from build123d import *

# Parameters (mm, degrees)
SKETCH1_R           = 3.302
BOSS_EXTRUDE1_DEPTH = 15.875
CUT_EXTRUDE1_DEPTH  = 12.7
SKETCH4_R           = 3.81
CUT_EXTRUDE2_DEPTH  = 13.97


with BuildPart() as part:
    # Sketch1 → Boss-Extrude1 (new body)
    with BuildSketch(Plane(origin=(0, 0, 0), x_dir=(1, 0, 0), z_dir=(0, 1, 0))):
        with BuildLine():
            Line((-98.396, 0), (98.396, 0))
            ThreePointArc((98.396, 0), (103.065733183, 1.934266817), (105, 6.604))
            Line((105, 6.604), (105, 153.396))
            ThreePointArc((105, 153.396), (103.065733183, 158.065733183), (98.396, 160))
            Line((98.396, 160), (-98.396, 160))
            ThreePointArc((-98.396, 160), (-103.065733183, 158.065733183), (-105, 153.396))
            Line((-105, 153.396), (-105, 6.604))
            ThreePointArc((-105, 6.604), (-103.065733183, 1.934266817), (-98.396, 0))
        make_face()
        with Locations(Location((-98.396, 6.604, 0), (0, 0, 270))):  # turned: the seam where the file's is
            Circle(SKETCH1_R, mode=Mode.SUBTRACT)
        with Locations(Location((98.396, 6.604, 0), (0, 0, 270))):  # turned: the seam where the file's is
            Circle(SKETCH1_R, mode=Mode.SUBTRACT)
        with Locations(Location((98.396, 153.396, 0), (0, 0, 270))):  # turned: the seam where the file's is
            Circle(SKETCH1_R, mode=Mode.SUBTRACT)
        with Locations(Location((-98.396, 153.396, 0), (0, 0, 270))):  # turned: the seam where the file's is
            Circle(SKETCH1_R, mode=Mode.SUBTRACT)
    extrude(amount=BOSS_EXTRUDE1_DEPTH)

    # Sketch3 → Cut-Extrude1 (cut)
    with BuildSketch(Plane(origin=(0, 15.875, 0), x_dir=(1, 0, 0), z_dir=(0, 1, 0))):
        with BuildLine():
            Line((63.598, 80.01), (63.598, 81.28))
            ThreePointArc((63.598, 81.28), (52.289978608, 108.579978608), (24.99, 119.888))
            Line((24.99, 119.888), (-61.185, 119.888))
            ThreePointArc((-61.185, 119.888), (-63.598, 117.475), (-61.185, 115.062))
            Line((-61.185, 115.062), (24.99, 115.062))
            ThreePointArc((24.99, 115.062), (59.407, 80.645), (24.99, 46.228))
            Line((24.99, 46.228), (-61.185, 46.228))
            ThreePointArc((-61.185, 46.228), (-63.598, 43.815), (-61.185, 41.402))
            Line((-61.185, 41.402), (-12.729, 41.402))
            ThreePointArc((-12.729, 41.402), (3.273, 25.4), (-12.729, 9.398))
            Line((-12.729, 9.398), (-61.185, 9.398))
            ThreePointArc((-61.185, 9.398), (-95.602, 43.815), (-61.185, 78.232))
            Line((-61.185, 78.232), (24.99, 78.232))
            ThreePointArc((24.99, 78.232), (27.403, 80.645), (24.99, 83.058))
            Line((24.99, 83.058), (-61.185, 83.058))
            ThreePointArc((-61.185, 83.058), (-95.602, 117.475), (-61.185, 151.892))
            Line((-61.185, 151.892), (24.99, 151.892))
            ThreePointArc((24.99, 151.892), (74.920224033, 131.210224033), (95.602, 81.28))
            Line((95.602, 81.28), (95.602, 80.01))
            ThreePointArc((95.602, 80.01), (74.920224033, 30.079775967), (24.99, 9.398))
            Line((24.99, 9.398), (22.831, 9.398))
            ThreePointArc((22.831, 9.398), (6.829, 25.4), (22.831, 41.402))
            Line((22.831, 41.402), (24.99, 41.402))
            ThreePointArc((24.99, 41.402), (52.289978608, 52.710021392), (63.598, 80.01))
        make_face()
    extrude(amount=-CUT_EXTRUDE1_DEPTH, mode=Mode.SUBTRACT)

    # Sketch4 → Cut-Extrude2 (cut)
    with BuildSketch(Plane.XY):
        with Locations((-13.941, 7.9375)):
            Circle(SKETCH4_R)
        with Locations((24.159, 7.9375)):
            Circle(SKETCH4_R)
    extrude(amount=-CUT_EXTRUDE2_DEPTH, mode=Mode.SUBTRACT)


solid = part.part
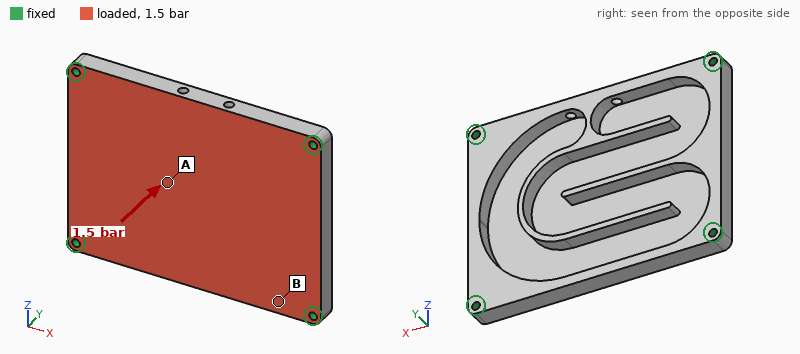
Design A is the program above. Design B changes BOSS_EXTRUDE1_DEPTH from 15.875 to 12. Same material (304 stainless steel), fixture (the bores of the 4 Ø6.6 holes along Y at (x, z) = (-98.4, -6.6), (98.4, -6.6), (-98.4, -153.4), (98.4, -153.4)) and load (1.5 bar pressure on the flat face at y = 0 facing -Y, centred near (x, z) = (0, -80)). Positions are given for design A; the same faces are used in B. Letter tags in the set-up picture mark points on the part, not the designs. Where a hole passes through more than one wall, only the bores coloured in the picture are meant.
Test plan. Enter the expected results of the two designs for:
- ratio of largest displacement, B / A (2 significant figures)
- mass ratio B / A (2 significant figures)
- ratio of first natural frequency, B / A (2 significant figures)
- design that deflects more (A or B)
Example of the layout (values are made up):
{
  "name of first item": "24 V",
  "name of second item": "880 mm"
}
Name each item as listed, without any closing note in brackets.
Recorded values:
{
  "ratio of largest displacement, B / A": "1.6",
  "mass ratio B / A": "0.82",
  "ratio of first natural frequency, B / A": "0.83",
  "design that deflects more": "B"
}
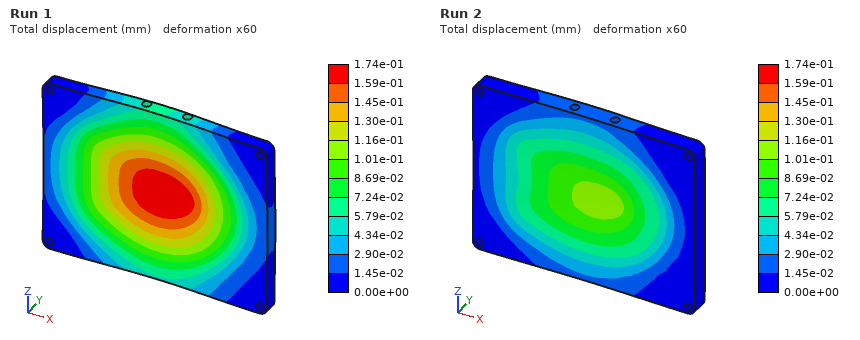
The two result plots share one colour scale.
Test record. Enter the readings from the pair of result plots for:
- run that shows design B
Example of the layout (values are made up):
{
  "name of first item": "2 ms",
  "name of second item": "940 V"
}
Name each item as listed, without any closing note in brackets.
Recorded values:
{
  "run that shows design B": "Run 1"
}
